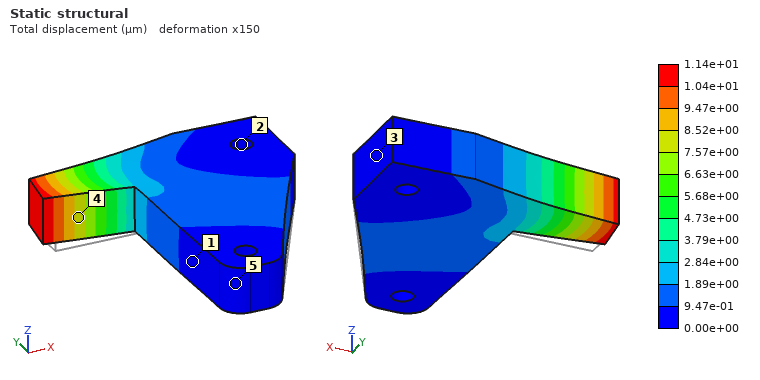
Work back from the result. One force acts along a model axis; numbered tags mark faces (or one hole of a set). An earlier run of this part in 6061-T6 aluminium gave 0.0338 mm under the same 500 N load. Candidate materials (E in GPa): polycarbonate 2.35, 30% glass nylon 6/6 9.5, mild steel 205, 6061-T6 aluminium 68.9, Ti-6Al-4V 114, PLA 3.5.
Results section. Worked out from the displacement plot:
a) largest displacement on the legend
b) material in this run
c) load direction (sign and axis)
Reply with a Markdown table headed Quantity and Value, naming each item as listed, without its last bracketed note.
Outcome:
| Quantity | Value |
|---|---|
| largest displacement on the legend | 1.14e+01 µm |
| material in this run | mild steel |
| load direction | +Y |
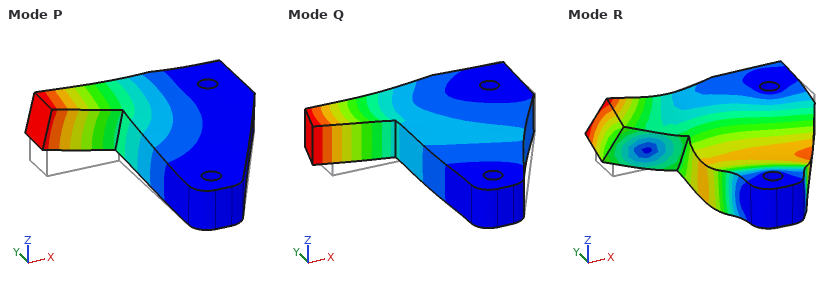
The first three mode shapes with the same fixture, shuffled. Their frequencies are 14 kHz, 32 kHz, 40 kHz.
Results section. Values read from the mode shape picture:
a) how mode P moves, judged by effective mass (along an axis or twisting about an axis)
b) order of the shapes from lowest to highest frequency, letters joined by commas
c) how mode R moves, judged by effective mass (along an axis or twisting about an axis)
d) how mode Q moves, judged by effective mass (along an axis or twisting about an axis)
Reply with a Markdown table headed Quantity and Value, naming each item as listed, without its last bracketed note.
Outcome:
| Quantity | Value |
|---|---|
| how mode P moves, judged by effective mass | along Z |
| order of the shapes from lowest to highest frequency, letters joined by commas | P, Q, R |
| how mode R moves, judged by effective mass | along Z |
| how mode Q moves, judged by effective mass | along Y |
